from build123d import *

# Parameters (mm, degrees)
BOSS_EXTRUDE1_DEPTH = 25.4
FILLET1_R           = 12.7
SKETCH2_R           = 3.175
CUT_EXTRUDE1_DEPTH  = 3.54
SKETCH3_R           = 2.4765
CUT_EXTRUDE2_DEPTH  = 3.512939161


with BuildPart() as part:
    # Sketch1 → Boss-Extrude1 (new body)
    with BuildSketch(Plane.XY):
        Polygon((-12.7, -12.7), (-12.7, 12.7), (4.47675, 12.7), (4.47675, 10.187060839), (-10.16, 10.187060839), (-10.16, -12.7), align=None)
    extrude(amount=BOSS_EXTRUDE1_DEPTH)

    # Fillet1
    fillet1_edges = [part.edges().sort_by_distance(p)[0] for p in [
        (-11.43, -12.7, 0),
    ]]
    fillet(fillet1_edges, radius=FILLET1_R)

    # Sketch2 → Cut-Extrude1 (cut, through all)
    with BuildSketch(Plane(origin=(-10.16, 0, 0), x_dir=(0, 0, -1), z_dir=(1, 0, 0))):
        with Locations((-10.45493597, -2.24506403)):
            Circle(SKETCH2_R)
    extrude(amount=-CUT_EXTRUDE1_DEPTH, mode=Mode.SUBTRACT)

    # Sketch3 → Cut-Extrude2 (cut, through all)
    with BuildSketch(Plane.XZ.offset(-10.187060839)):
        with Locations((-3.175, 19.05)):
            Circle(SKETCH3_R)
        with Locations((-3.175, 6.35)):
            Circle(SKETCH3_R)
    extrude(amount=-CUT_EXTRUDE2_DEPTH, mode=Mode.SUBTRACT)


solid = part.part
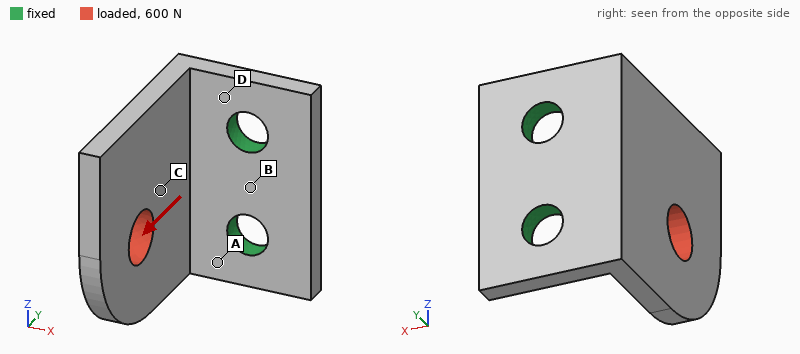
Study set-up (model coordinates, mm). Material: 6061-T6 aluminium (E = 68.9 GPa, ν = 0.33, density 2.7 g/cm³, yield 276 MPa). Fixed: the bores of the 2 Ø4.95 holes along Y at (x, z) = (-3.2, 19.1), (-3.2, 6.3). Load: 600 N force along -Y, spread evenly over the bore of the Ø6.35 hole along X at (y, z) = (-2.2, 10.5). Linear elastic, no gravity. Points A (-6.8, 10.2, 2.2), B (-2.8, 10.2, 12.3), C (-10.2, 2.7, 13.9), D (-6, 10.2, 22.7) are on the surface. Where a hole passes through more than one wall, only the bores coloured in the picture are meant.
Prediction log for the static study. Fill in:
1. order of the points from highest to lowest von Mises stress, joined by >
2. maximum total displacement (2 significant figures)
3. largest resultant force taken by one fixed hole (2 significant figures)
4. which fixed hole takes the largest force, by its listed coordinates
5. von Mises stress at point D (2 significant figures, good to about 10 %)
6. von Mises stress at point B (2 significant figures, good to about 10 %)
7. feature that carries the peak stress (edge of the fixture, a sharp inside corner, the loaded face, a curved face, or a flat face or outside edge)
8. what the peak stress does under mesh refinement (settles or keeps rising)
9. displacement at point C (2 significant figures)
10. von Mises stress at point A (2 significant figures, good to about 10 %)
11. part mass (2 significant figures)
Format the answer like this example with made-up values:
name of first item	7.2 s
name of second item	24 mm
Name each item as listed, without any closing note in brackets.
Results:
order of the points from highest to lowest von Mises stress, joined by >	A > D > B > C
maximum total displacement	0.14 mm
largest resultant force taken by one fixed hole	380 N
which fixed hole takes the largest force, by its listed coordinates	(-3.2, 6.3)
von Mises stress at point D	60 MPa
von Mises stress at point B	31 MPa
feature that carries the peak stress	edge of the fixture
what the peak stress does under mesh refinement	keeps rising
displacement at point C	0.054 mm
von Mises stress at point A	85 MPa
part mass	6.2 g
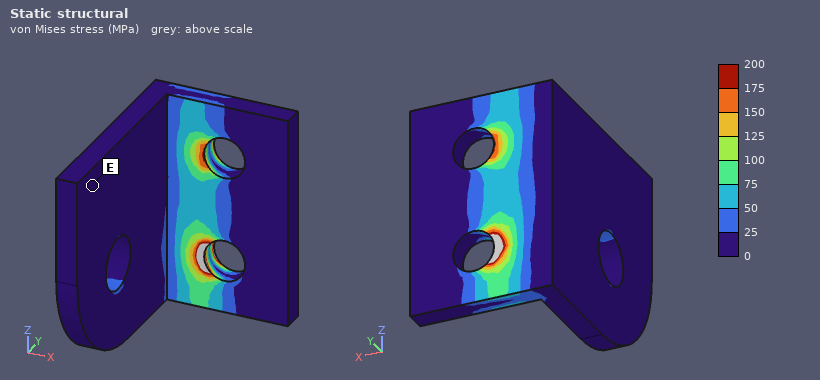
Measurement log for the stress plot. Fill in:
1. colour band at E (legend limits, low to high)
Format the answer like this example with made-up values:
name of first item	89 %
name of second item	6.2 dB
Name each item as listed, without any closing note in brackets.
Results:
colour band at E	0 to 25 MPa
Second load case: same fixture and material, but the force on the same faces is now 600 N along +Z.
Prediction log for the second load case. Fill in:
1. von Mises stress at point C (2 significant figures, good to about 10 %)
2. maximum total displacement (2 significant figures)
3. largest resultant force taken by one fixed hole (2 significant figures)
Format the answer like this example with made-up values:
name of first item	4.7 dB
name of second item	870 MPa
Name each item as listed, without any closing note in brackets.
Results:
von Mises stress at point C	39 MPa
maximum total displacement	0.13 mm
largest resultant force taken by one fixed hole	640 N
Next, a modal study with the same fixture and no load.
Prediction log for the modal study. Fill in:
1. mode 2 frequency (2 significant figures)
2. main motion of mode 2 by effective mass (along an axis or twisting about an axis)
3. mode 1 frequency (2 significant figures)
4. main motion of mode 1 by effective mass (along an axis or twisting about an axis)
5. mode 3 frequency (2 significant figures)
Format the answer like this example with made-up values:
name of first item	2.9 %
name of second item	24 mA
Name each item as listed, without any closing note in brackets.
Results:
mode 2 frequency	6700 Hz
main motion of mode 2 by effective mass	along Z
mode 1 frequency	2800 Hz
main motion of mode 1 by effective mass	along X
mode 3 frequency	9500 Hz
